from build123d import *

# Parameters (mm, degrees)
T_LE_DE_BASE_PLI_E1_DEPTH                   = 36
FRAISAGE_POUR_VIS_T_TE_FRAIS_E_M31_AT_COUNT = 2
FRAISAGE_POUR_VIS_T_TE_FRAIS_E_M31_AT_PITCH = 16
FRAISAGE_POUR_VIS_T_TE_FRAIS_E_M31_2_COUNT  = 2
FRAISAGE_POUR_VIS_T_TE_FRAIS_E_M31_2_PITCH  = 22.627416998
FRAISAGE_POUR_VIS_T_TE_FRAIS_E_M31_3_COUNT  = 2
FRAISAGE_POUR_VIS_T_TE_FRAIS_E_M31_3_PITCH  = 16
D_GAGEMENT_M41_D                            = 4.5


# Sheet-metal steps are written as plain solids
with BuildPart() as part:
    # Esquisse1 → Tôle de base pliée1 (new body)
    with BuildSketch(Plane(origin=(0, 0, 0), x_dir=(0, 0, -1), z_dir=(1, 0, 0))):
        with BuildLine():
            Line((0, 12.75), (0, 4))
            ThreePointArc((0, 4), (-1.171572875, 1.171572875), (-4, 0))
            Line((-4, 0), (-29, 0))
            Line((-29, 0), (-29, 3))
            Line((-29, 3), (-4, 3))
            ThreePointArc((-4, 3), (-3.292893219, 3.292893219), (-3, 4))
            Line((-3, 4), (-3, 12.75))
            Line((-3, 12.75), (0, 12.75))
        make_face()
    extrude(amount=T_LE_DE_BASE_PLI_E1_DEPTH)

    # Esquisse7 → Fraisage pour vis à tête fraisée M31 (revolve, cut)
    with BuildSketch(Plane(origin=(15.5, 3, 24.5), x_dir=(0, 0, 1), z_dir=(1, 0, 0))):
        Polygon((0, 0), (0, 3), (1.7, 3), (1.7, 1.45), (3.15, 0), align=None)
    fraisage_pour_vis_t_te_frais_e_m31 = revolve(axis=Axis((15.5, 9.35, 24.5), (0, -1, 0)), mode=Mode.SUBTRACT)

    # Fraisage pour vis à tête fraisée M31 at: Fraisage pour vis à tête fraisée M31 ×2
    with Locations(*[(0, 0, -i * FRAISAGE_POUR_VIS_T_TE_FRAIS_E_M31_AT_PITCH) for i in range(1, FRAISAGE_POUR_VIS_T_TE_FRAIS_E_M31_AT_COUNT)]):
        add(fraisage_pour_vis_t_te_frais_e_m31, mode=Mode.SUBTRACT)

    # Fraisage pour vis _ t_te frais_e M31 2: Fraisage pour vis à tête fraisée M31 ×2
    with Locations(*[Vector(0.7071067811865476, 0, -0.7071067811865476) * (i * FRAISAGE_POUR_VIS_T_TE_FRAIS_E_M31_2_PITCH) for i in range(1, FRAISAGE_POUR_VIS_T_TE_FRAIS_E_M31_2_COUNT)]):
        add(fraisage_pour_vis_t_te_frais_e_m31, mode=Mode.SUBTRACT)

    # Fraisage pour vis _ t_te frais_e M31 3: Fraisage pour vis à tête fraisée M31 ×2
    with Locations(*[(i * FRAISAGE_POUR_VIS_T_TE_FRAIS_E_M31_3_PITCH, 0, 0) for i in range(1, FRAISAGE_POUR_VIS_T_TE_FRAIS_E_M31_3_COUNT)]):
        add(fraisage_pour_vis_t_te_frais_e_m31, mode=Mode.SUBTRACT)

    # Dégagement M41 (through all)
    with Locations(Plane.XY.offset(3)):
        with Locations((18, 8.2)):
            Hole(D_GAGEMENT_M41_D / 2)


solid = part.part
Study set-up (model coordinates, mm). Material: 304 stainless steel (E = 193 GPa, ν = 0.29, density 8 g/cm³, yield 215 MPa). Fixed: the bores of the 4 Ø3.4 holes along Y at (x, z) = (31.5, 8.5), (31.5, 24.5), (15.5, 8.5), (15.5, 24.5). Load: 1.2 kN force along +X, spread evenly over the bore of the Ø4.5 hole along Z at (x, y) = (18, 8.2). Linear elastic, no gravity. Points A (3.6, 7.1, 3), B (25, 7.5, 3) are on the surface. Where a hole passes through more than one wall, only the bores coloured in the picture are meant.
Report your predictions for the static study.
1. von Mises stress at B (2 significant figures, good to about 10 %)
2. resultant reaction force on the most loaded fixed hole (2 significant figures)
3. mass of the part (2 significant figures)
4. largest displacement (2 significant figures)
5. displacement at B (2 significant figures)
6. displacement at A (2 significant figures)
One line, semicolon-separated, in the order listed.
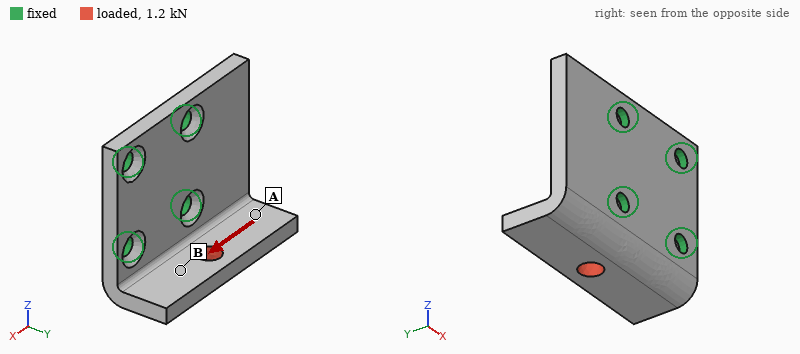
53 MPa; 890 N; 31 g; 27 µm; 8.2 µm; 18 µm
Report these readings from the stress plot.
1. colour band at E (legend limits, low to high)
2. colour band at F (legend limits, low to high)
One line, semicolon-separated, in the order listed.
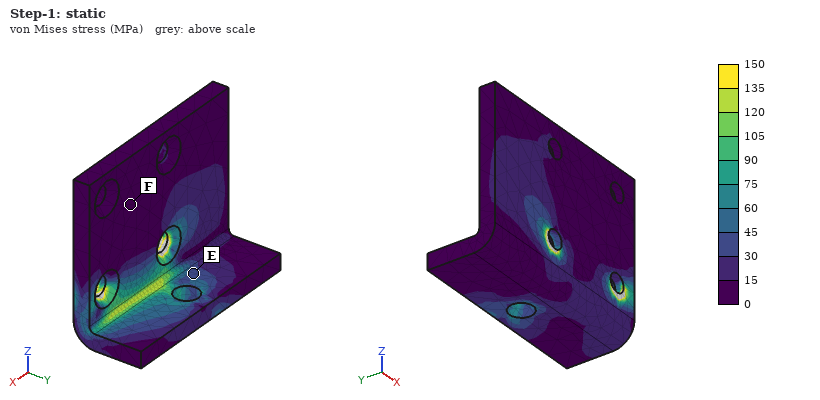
30 to 45 MPa; 0 to 15 MPa
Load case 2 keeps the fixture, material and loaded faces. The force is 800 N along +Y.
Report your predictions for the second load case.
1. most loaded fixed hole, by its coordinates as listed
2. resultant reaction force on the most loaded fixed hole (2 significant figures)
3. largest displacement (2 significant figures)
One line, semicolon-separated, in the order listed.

(15.5, 8.5); 790 N; 32 µm
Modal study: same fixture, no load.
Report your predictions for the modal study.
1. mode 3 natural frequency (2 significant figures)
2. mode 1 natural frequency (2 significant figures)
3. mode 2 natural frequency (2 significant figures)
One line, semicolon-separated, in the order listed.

11 kHz; 7700 Hz; 9400 Hz
